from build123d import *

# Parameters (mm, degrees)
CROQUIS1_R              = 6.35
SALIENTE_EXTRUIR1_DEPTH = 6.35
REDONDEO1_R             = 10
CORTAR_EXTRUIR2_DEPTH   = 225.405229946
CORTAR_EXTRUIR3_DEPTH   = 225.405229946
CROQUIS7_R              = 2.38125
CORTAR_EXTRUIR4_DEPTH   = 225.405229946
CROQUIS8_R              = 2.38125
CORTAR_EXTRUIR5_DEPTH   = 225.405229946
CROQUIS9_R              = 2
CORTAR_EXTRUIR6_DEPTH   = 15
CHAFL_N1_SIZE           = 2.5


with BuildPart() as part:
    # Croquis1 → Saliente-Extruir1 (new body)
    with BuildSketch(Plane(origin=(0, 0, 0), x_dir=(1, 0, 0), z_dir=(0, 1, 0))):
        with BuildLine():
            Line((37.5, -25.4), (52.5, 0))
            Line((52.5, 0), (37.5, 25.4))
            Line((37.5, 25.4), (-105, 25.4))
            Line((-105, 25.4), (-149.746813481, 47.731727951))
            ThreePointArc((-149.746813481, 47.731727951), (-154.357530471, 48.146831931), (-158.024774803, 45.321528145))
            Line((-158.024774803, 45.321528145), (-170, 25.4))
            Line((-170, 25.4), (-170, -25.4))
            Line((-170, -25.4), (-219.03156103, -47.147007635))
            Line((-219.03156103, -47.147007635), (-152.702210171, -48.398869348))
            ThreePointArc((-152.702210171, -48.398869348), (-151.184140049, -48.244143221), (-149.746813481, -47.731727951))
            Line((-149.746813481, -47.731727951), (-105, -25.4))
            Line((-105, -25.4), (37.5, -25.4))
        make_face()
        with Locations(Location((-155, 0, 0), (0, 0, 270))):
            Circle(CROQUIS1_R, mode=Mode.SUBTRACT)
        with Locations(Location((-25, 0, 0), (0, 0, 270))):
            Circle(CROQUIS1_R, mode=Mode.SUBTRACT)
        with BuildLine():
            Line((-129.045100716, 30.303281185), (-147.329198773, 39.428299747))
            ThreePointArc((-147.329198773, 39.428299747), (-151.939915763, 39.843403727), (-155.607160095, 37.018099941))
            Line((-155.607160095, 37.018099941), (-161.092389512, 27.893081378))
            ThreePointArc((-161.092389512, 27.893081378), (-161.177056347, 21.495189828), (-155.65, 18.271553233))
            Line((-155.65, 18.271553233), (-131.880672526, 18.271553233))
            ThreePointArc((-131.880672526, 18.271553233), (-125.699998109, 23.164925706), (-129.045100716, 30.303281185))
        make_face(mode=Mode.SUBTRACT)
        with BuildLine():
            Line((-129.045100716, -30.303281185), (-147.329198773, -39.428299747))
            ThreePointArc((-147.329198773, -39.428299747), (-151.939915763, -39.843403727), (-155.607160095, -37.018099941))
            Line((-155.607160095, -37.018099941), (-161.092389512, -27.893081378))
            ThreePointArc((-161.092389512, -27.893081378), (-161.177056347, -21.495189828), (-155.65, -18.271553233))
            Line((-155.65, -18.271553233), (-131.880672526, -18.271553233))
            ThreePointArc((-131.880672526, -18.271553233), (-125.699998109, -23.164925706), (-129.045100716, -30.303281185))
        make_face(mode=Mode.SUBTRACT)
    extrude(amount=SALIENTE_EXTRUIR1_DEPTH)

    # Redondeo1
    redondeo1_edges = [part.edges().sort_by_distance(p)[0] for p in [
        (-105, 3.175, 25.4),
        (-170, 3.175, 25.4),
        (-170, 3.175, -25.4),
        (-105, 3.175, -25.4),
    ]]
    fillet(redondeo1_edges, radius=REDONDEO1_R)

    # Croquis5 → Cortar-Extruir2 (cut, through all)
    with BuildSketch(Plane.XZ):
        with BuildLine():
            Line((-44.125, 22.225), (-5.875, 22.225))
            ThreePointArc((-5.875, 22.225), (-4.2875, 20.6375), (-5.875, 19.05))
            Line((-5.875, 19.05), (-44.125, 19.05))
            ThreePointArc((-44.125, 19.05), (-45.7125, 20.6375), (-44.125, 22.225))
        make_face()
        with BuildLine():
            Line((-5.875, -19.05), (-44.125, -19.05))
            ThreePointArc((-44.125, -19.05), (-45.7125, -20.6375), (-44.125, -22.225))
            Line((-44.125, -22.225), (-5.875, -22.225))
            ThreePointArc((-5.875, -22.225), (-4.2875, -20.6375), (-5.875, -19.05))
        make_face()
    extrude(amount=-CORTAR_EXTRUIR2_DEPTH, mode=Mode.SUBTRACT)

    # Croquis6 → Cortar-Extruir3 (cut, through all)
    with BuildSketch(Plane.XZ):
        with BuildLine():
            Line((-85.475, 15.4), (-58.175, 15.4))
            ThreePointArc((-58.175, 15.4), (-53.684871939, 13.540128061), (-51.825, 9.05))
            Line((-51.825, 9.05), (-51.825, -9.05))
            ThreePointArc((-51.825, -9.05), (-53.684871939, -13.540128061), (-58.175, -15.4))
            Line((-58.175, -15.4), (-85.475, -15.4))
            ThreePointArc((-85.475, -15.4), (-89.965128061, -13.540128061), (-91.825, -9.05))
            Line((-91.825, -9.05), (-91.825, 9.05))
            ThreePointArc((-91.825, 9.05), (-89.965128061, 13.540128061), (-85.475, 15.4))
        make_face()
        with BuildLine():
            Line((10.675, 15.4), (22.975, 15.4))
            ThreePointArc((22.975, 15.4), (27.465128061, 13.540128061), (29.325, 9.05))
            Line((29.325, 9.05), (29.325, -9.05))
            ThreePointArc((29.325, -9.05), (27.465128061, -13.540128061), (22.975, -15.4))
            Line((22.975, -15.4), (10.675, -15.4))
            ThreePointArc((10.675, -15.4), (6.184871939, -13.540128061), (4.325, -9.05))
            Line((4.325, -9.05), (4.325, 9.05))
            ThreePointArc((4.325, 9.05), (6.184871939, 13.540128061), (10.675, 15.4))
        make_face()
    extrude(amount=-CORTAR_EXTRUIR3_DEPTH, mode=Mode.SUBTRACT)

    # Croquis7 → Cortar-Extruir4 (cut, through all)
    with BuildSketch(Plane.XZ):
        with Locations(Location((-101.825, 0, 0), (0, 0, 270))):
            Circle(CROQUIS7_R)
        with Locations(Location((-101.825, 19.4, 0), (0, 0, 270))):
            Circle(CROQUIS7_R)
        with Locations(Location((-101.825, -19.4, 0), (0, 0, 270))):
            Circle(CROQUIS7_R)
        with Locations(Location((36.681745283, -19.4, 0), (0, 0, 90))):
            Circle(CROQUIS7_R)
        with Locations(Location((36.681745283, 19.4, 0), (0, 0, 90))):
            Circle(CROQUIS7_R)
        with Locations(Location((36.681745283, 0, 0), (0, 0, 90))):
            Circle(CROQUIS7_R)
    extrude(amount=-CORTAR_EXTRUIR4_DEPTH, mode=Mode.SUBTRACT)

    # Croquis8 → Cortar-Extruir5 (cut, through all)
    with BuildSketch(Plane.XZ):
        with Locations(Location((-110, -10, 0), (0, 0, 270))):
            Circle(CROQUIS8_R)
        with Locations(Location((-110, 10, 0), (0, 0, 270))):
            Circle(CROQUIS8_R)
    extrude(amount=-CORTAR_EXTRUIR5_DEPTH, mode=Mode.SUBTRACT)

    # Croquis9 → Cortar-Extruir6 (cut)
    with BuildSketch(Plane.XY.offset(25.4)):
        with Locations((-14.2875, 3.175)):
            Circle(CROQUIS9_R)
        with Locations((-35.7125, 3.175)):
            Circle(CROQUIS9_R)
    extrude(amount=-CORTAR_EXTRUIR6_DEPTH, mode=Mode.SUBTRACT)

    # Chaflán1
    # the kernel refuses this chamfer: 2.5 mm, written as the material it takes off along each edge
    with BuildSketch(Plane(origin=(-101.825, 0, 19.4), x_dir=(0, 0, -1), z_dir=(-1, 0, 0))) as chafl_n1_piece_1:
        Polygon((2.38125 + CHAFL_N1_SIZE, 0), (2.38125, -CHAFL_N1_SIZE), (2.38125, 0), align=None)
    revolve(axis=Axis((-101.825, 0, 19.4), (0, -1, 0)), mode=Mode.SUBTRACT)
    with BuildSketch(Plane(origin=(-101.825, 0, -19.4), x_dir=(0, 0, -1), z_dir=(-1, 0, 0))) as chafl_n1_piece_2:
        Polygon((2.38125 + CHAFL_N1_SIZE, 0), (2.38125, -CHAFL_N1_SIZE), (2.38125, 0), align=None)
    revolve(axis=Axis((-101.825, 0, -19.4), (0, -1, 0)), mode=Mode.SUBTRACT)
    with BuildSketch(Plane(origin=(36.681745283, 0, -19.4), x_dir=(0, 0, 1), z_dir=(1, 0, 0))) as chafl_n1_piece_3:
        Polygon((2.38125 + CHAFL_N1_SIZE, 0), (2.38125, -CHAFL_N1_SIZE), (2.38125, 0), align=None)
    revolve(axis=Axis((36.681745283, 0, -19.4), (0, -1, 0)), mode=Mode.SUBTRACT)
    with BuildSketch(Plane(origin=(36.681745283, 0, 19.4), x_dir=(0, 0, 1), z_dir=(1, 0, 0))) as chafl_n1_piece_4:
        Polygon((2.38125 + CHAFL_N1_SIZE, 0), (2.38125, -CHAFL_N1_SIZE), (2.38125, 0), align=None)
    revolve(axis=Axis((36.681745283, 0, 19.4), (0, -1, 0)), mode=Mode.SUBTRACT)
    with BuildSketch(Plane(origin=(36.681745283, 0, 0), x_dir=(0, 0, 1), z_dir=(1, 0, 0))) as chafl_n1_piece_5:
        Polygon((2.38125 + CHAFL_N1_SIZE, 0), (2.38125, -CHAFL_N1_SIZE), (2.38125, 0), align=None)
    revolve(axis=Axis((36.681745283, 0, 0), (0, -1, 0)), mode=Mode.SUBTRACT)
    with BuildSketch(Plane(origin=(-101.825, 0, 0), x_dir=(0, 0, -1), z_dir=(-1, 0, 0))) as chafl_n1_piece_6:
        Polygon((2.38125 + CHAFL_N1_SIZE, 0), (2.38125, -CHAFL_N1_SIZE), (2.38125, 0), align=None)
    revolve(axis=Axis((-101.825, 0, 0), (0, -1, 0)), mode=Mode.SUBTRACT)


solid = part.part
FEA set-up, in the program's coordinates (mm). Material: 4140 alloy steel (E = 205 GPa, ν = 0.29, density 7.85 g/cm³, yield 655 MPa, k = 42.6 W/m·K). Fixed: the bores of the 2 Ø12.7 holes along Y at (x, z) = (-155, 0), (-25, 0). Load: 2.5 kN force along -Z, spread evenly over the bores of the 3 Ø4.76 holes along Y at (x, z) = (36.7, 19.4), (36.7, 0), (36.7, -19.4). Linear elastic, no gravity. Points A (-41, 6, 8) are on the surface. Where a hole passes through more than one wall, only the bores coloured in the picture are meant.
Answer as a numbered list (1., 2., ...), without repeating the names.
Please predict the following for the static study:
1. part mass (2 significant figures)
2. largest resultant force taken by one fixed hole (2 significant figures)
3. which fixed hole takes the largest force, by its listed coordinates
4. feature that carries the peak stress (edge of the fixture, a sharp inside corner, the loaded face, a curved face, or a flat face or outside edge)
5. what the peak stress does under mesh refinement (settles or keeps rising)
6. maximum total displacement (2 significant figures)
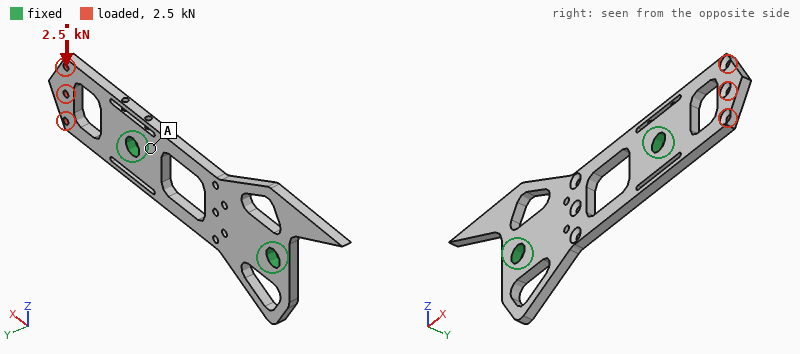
1. 470 g
2. 2.9 kN
3. (-25, 0)
4. a sharp inside corner
5. keeps rising
6. 0.10 mm
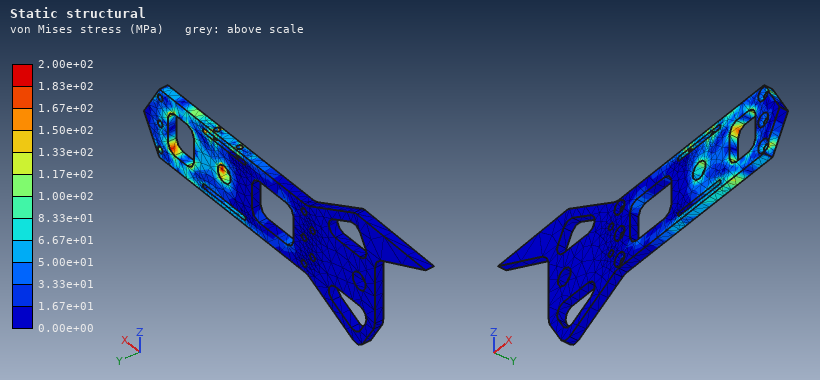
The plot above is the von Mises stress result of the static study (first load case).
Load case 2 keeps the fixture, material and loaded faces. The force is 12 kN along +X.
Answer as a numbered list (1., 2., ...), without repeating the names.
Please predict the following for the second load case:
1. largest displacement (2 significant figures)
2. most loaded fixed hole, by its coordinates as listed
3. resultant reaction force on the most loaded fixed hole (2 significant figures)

1. 0.32 mm
2. (-25, 0)
3. 11 kN
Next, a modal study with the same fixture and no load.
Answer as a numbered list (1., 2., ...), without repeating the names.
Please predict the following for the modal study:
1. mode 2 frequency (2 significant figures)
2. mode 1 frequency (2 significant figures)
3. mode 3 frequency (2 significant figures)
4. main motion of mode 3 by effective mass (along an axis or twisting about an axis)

1. 1300 Hz
2. 1100 Hz
3. 2000 Hz
4. along Y
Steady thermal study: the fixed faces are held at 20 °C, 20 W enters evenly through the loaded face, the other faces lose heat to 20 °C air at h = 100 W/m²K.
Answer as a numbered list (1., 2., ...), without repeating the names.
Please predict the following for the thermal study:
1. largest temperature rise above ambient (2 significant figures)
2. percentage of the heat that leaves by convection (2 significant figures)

1. 59 K
2. 86 %
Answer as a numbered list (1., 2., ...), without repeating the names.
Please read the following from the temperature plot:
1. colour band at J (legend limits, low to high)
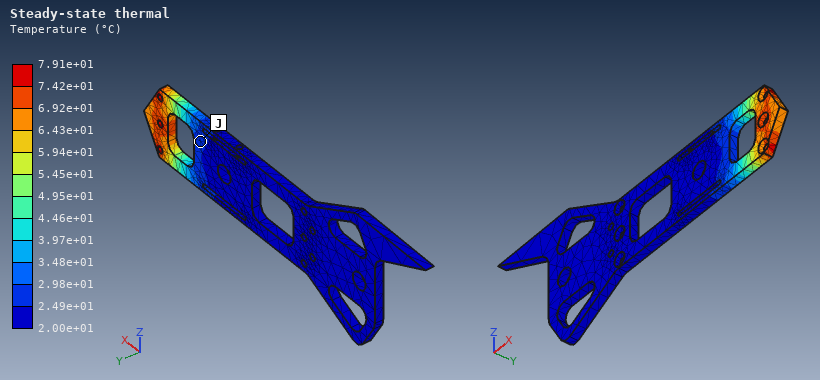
1. 2.49e+01 to 2.98e+01 °C
